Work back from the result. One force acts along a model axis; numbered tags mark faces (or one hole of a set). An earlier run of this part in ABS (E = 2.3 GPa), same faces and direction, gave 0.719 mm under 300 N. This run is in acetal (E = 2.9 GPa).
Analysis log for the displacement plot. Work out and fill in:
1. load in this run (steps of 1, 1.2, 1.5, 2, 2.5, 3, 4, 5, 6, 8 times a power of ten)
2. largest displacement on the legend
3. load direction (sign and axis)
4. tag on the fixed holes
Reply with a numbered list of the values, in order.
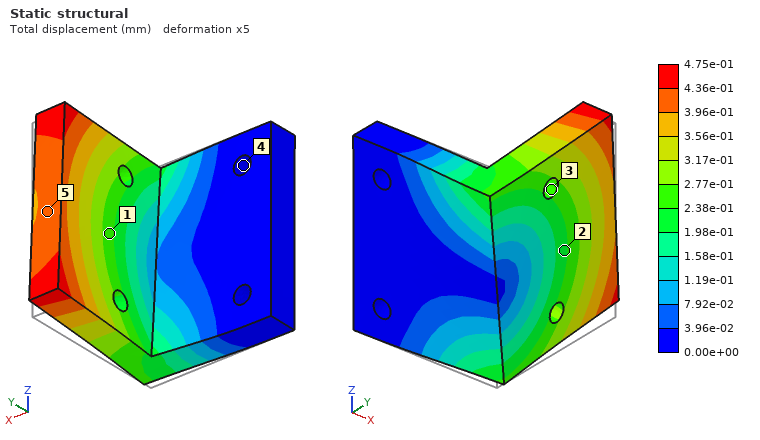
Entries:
1. 250 N
2. 4.75e-01 mm
3. +Z
4. 4
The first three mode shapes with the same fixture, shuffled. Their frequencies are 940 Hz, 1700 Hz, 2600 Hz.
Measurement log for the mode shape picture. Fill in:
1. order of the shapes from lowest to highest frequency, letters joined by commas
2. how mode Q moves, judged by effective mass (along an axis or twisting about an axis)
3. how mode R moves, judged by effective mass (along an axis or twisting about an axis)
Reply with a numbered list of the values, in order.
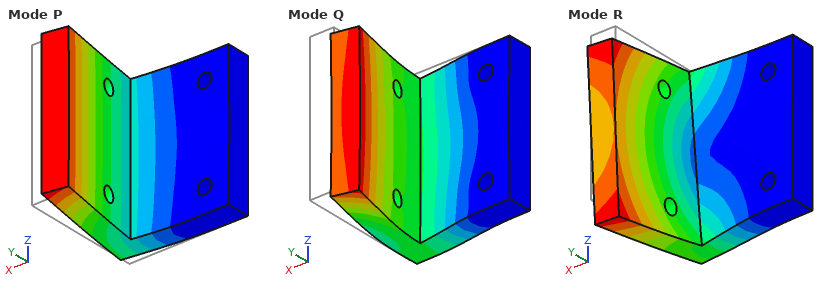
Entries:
1. P, R, Q
2. along Y
3. along Z
